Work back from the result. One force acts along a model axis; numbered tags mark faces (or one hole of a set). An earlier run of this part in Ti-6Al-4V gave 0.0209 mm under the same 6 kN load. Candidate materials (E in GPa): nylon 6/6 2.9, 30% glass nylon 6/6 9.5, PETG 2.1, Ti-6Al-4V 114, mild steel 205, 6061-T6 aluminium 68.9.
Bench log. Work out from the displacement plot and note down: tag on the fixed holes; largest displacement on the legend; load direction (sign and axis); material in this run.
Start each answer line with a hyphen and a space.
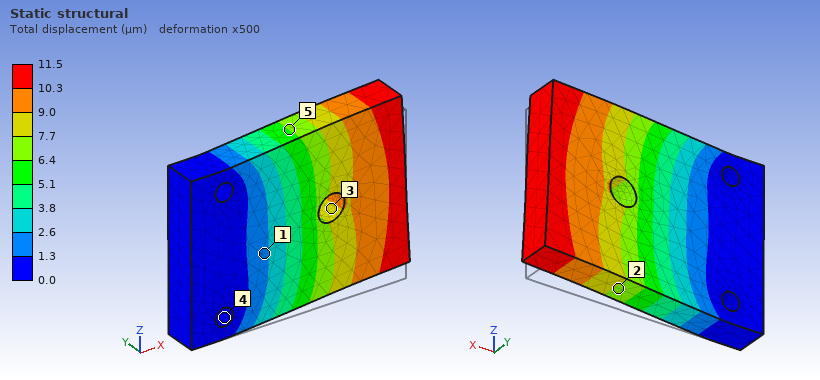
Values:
- 4
- 11.5 µm
- +Z
- mild steel
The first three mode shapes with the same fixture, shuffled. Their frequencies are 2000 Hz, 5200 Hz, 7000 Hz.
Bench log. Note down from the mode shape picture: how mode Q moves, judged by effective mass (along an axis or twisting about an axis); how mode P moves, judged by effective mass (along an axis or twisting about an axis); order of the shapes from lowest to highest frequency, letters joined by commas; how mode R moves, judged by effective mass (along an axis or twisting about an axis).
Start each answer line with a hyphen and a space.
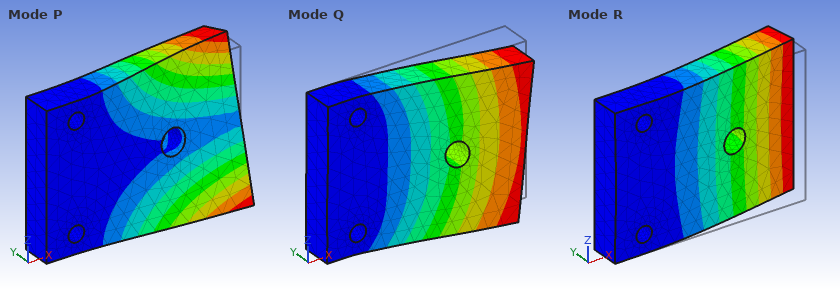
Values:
- along Z
- twisting about X
- R, P, Q
- along Y
